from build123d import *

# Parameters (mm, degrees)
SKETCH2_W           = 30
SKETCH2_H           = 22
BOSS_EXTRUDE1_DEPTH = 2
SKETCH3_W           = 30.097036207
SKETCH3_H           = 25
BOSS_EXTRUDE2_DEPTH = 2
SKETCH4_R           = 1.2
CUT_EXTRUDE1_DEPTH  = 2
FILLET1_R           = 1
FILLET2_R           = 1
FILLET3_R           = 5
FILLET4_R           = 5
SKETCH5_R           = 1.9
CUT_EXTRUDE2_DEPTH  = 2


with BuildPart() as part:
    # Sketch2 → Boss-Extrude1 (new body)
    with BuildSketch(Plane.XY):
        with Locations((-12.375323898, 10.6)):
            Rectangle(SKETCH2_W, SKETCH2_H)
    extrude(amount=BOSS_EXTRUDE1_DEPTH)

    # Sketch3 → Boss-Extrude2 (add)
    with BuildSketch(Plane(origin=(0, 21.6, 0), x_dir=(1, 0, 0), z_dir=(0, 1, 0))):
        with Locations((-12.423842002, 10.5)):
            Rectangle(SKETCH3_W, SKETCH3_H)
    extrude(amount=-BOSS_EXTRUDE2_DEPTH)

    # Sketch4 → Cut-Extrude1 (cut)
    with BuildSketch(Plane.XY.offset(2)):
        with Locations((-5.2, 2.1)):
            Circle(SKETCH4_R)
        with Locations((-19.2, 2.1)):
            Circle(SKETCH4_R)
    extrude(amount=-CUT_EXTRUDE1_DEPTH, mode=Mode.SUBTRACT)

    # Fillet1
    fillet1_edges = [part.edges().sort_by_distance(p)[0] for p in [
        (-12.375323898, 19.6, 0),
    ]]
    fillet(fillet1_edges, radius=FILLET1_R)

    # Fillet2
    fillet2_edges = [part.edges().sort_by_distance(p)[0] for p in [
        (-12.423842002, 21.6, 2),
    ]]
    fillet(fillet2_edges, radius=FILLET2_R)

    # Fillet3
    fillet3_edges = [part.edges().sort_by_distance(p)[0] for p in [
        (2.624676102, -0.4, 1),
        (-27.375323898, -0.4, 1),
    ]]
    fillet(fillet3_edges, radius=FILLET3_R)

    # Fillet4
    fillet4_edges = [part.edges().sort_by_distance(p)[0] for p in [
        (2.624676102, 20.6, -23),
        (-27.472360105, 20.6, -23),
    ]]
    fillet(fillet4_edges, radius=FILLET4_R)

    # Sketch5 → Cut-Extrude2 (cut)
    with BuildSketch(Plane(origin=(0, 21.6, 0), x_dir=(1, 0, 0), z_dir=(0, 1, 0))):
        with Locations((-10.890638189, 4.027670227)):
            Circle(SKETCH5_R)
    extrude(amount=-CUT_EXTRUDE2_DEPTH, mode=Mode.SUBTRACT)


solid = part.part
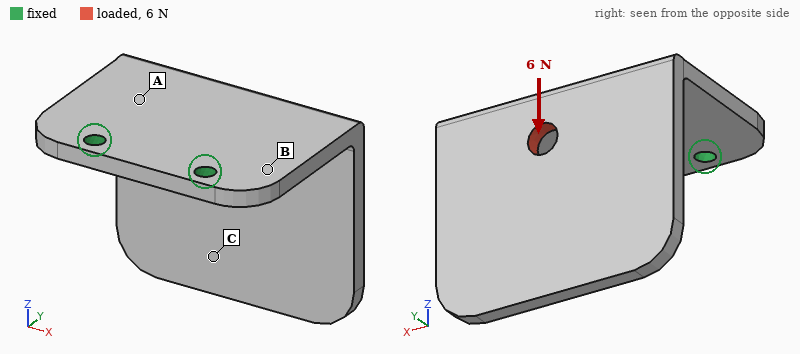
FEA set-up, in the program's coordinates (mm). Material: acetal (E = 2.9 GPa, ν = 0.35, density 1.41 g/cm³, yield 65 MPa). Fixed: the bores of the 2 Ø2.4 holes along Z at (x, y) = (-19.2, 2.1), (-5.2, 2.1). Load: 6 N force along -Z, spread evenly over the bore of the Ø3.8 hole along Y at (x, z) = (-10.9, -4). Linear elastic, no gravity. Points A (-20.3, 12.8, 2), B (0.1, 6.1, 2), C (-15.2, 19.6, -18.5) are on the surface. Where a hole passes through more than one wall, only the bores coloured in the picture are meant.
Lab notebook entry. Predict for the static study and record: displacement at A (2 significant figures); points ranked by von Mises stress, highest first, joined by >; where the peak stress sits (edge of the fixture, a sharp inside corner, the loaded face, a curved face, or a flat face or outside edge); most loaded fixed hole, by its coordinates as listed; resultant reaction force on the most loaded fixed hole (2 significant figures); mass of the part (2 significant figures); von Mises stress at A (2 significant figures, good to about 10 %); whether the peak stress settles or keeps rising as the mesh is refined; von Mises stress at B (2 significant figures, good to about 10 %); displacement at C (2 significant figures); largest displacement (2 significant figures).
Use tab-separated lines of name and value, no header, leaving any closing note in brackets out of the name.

displacement at A	0.093 mm
points ranked by von Mises stress, highest first, joined by >	B > A > C
where the peak stress sits	edge of the fixture
most loaded fixed hole, by its coordinates as listed	(-5.2, 2.1)
resultant reaction force on the most loaded fixed hole	3.4 N
mass of the part	3.7 g
von Mises stress at A	2.0 MPa
whether the peak stress settles or keeps rising as the mesh is refined	keeps rising
von Mises stress at B	3.8 MPa
displacement at C	0.40 mm
largest displacement	0.50 mm
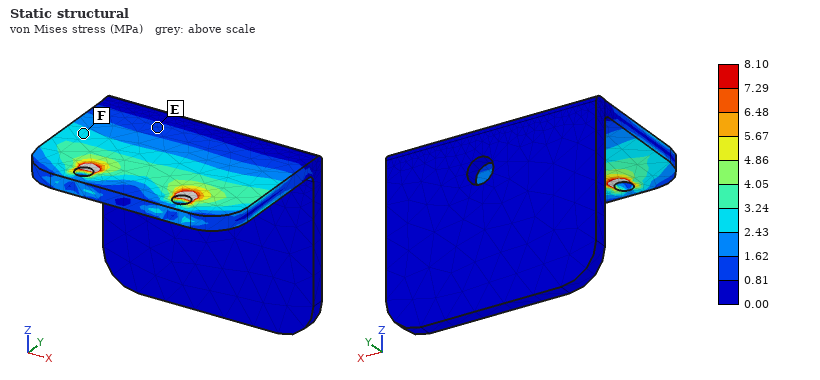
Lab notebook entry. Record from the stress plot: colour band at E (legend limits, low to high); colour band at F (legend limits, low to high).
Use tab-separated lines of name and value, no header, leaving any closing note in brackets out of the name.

colour band at E	0.81 to 1.62 MPa
colour band at F	2.43 to 3.24 MPa
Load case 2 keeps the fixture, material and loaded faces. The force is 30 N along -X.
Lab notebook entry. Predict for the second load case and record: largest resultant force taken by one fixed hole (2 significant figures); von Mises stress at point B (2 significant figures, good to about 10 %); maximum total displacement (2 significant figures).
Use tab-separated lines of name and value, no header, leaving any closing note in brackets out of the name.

largest resultant force taken by one fixed hole	39 N
von Mises stress at point B	4.4 MPa
maximum total displacement	0.49 mm
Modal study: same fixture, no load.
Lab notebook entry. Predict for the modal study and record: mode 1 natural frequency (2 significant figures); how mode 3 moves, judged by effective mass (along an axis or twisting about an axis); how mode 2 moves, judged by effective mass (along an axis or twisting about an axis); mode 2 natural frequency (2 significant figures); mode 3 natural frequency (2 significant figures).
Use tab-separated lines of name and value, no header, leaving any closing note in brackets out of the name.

mode 1 natural frequency	350 Hz
how mode 3 moves, judged by effective mass	along Z
how mode 2 moves, judged by effective mass	along X
mode 2 natural frequency	610 Hz
mode 3 natural frequency	980 Hz
